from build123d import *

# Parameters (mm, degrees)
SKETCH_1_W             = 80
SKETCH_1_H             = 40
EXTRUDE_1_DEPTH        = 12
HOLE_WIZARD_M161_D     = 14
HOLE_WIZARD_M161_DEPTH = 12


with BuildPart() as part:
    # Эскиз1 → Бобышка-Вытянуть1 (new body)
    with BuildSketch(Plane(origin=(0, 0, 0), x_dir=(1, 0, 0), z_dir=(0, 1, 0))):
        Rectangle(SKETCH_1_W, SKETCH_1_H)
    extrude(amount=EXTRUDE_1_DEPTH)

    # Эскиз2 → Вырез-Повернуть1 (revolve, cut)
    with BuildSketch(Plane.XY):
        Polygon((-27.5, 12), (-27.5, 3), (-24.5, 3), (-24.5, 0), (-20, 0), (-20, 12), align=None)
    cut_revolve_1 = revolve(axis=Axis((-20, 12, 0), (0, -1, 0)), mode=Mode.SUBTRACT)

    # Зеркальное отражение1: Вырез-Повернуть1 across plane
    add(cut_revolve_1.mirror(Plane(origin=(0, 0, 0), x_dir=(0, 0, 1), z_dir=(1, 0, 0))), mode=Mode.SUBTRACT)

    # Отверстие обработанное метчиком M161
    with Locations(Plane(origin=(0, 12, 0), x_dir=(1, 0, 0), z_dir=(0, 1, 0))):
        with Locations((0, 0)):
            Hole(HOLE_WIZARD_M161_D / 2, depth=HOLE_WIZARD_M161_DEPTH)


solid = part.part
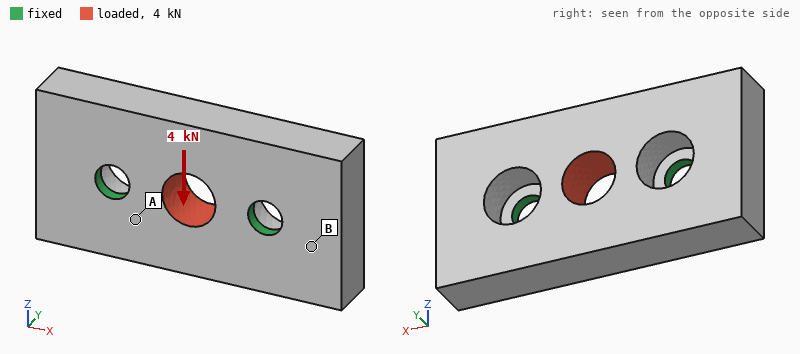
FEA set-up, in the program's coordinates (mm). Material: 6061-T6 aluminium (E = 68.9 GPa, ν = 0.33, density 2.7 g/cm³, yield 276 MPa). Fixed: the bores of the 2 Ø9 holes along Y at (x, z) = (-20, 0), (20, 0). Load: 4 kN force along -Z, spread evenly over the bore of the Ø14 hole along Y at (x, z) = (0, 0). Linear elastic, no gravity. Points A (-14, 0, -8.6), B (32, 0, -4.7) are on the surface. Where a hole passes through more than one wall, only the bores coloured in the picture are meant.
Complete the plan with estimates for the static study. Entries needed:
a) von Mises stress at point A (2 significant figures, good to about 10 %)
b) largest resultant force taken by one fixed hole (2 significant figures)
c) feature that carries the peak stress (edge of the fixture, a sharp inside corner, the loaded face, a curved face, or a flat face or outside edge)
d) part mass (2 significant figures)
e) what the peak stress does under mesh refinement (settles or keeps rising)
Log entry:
26 MPa
2.0 kN
edge of the fixture
89 g
keeps rising
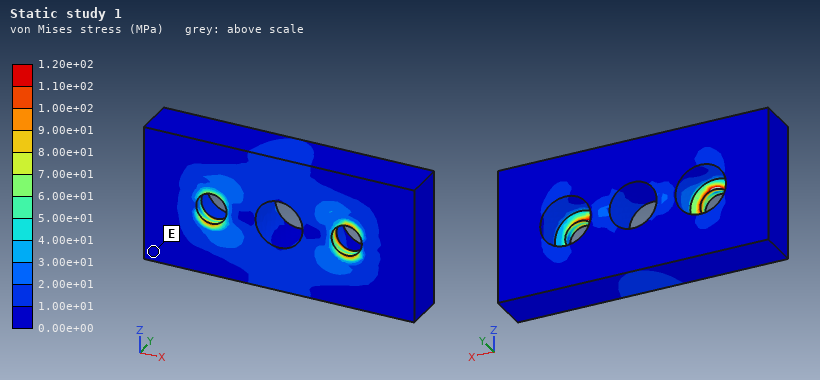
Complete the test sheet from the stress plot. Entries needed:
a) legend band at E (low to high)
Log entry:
0.00e+00 to 1.00e+01 MPa
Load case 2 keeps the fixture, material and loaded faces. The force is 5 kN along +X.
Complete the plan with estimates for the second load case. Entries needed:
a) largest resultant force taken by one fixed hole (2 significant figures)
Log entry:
2.6 kN
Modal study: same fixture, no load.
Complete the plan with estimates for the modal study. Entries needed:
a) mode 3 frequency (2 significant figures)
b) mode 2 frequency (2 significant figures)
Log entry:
9700 Hz
9100 Hz
